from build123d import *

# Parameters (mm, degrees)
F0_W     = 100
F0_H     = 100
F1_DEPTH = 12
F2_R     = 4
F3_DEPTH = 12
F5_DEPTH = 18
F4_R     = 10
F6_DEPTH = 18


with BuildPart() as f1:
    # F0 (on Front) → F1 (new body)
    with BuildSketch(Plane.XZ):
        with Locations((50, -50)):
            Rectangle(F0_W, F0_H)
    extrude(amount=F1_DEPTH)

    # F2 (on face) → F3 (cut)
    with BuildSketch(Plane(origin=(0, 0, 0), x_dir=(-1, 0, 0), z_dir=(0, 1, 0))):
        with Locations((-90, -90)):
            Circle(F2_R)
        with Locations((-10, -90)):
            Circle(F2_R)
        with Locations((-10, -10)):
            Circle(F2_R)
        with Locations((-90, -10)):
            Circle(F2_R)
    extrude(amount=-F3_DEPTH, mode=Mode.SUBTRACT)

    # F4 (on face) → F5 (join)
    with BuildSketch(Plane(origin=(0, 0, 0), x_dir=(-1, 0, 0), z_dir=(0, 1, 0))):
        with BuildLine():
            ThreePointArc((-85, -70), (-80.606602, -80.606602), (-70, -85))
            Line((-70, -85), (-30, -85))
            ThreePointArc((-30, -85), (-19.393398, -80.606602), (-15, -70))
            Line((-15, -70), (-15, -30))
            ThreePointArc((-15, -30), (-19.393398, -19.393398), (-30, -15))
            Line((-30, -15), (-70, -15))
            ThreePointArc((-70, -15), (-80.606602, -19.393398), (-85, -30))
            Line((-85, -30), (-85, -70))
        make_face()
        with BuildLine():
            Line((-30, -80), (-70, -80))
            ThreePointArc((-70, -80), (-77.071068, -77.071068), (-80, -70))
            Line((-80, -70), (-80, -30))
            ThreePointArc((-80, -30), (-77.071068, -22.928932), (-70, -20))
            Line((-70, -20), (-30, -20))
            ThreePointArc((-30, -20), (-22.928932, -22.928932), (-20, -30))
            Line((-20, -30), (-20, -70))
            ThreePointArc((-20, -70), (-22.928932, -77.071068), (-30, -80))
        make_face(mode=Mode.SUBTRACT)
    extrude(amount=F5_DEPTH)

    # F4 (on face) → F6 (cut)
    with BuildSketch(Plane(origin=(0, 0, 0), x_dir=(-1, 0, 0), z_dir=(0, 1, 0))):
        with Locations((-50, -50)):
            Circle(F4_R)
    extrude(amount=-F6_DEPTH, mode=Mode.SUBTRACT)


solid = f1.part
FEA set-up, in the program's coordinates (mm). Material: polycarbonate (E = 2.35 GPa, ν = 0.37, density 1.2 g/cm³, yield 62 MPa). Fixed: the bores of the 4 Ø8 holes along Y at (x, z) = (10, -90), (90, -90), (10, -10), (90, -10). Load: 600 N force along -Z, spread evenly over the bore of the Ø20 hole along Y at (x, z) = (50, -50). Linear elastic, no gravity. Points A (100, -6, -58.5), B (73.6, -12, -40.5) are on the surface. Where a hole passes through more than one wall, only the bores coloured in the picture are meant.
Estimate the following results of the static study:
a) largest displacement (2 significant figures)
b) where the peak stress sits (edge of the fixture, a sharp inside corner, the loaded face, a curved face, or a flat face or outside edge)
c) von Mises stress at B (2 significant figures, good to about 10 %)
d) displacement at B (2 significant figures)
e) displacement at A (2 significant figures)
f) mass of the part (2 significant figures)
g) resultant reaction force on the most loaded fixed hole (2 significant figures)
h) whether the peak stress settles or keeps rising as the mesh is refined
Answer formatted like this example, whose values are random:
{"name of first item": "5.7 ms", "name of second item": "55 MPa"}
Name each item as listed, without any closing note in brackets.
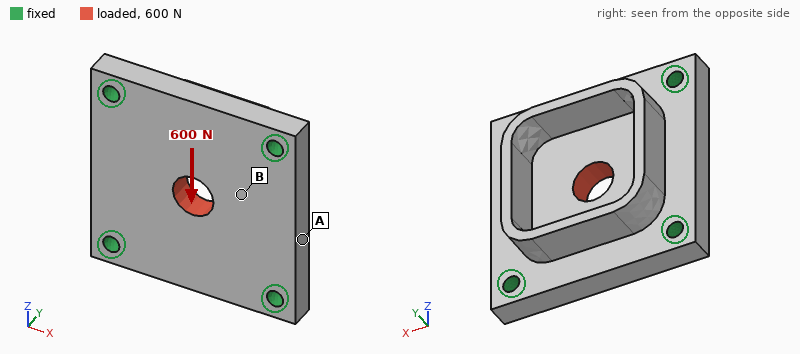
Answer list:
{"largest displacement": "16 µm", "where the peak stress sits": "edge of the fixture", "von Mises stress at B": "0.45 MPa", "displacement at B": "7.6 µm", "displacement at A": "2.9 µm", "mass of the part": "160 g", "resultant reaction force on the most loaded fixed hole": "170 N", "whether the peak stress settles or keeps rising as the mesh is refined": "keeps rising"}
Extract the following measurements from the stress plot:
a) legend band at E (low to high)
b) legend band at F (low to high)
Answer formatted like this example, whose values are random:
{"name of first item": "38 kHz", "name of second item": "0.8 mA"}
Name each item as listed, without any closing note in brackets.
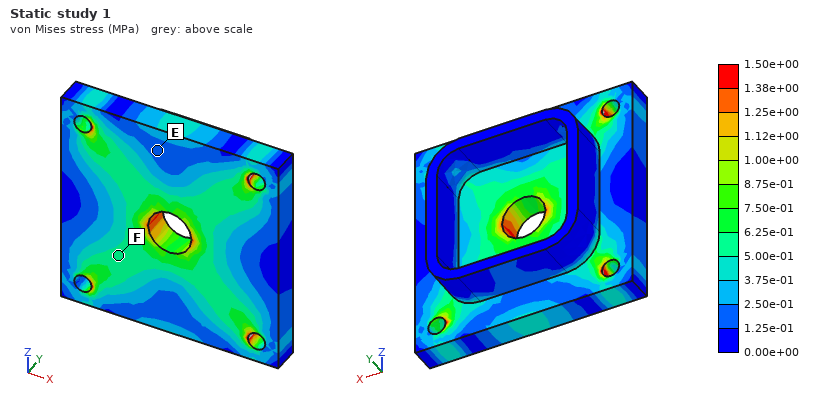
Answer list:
{"legend band at E": "1.25e-01 to 2.50e-01 MPa", "legend band at F": "5.00e-01 to 6.25e-01 MPa"}
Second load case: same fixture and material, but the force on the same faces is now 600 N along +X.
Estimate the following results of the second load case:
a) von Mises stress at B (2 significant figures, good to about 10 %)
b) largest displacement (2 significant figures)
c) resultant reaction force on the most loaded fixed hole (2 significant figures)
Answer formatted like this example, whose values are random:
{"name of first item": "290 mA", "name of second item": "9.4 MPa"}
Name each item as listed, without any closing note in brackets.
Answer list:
{"von Mises stress at B": "0.47 MPa", "largest displacement": "16 µm", "resultant reaction force on the most loaded fixed hole": "170 N"}
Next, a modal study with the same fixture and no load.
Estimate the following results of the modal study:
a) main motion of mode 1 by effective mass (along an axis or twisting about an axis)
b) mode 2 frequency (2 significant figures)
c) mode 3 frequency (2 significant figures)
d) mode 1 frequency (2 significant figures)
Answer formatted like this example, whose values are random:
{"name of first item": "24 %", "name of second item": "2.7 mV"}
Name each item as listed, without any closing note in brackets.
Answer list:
{"main motion of mode 1 by effective mass": "along Y", "mode 2 frequency": "2700 Hz", "mode 3 frequency": "2700 Hz", "mode 1 frequency": "1900 Hz"}
